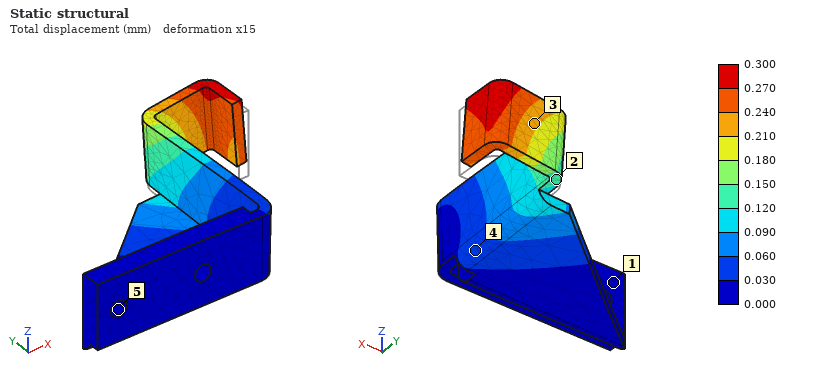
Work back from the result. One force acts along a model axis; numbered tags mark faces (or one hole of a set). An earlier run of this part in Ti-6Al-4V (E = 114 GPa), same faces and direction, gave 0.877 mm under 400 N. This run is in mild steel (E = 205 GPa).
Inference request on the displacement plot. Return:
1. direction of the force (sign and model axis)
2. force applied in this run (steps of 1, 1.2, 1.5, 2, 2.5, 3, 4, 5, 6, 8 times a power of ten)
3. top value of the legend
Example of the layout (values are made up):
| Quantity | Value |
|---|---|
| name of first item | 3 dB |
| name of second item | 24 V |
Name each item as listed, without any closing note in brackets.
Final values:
| Quantity | Value |
|---|---|
| direction of the force | +Z |
| force applied in this run | 250 N |
| top value of the legend | 0.300 mm |
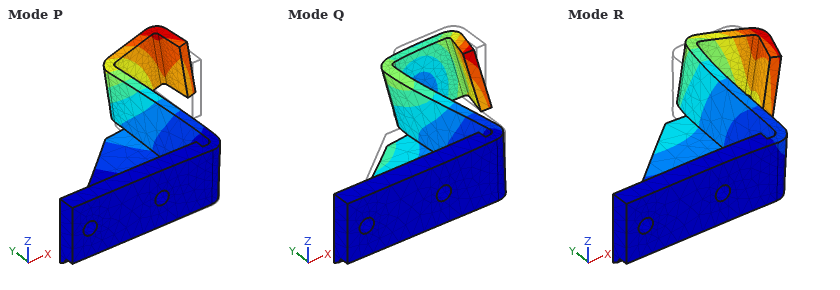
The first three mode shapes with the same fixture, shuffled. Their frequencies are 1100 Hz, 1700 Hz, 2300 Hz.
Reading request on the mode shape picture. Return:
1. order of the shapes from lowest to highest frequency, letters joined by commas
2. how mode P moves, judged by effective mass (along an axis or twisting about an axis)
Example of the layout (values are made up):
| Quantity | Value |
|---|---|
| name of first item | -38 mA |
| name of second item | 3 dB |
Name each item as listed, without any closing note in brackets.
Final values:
| Quantity | Value |
|---|---|
| order of the shapes from lowest to highest frequency, letters joined by commas | P, R, Q |
| how mode P moves, judged by effective mass | along Z |
